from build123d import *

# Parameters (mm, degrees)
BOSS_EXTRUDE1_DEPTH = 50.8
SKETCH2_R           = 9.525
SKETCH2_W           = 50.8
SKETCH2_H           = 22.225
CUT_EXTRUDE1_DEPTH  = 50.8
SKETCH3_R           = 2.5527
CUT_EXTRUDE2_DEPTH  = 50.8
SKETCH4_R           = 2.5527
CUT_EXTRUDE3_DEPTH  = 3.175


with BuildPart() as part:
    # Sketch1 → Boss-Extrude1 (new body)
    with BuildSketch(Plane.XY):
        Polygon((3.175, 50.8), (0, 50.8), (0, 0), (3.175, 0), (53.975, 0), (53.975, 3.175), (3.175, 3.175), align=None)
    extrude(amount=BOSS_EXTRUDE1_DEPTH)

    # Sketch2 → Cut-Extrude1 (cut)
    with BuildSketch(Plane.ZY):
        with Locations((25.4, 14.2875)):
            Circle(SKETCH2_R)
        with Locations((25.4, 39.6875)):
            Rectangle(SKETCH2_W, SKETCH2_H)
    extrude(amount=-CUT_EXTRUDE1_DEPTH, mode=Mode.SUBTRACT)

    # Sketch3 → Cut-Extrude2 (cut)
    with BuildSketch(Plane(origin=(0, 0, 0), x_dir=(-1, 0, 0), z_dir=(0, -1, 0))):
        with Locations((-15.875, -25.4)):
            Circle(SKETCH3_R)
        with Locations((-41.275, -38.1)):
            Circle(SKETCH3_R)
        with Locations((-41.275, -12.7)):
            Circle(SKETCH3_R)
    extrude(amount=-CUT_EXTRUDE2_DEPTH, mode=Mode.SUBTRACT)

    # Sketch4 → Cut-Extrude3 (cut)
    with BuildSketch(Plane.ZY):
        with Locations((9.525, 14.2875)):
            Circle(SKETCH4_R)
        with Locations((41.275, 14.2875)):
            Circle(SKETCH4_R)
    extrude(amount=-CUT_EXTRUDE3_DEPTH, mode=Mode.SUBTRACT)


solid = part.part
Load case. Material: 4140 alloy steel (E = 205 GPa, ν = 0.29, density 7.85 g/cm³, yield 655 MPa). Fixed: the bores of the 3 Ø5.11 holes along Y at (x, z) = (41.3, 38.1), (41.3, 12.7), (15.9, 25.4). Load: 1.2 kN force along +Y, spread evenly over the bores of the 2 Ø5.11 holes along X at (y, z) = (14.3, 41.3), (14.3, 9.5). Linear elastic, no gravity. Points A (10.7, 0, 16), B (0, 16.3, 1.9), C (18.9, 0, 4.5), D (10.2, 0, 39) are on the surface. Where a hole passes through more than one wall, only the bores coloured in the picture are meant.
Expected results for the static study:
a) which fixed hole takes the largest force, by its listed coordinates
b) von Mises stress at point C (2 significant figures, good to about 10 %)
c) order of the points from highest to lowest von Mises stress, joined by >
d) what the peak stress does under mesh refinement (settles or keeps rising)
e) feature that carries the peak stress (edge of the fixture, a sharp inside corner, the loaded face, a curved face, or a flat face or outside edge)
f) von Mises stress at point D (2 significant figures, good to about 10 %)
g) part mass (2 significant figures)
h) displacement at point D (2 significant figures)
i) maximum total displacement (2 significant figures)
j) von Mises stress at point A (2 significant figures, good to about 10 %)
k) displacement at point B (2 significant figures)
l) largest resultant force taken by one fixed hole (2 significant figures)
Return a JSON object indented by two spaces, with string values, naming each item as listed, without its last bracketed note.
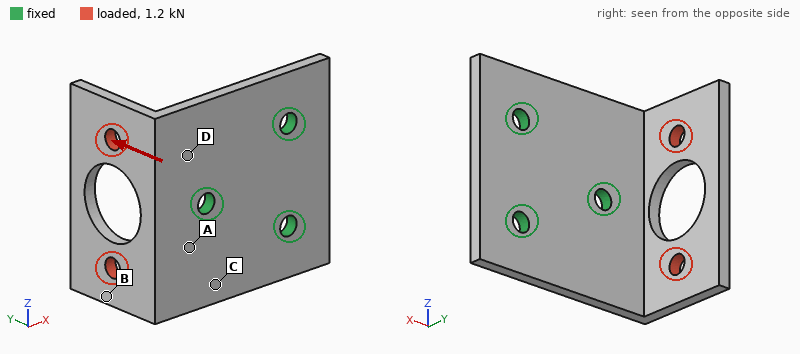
{
  "which fixed hole takes the largest force, by its listed coordinates": "(15.9, 25.4)",
  "von Mises stress at point C": "59 MPa",
  "order of the points from highest to lowest von Mises stress, joined by >": "A > D > C > B",
  "what the peak stress does under mesh refinement": "keeps rising",
  "feature that carries the peak stress": "edge of the fixture",
  "von Mises stress at point D": "85 MPa",
  "part mass": "91 g",
  "displacement at point D": "0.026 mm",
  "maximum total displacement": "0.15 mm",
  "von Mises stress at point A": "120 MPa",
  "displacement at point B": "0.10 mm",
  "largest resultant force taken by one fixed hole": "1.4 kN"
}
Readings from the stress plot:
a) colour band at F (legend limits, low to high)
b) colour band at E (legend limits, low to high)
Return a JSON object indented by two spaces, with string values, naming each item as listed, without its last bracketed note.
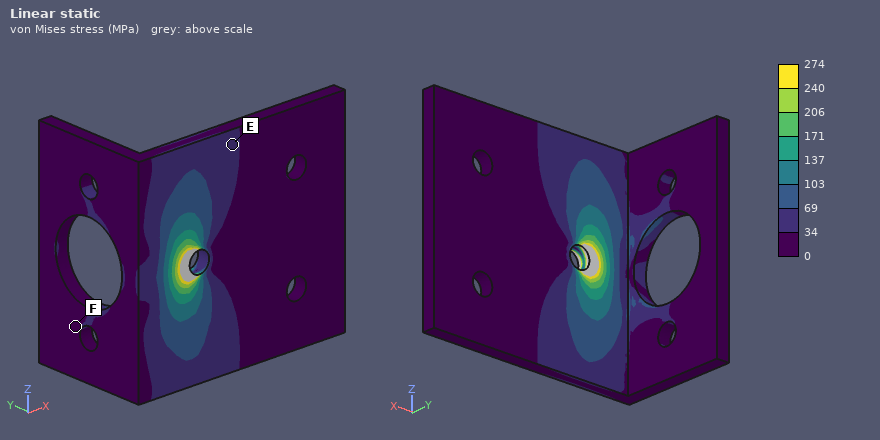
{
  "colour band at F": "0 to 34 MPa",
  "colour band at E": "34 to 69 MPa"
}
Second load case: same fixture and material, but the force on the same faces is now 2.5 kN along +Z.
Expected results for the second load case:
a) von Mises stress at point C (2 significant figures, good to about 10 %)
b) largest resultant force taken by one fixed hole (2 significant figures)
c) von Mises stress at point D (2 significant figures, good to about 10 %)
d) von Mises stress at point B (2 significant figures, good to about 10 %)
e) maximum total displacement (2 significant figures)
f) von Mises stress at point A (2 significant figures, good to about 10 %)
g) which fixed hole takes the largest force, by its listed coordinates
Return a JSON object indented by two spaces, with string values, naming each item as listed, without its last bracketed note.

{
  "von Mises stress at point C": "160 MPa",
  "largest resultant force taken by one fixed hole": "2.9 kN",
  "von Mises stress at point D": "110 MPa",
  "von Mises stress at point B": "86 MPa",
  "maximum total displacement": "0.41 mm",
  "von Mises stress at point A": "140 MPa",
  "which fixed hole takes the largest force, by its listed coordinates": "(15.9, 25.4)"
}
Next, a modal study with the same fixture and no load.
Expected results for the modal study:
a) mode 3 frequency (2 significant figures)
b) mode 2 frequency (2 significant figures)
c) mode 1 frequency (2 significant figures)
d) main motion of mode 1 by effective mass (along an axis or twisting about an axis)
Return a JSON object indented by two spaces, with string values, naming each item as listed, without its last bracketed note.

{
  "mode 3 frequency": "4200 Hz",
  "mode 2 frequency": "2100 Hz",
  "mode 1 frequency": "1900 Hz",
  "main motion of mode 1 by effective mass": "along X"
}
